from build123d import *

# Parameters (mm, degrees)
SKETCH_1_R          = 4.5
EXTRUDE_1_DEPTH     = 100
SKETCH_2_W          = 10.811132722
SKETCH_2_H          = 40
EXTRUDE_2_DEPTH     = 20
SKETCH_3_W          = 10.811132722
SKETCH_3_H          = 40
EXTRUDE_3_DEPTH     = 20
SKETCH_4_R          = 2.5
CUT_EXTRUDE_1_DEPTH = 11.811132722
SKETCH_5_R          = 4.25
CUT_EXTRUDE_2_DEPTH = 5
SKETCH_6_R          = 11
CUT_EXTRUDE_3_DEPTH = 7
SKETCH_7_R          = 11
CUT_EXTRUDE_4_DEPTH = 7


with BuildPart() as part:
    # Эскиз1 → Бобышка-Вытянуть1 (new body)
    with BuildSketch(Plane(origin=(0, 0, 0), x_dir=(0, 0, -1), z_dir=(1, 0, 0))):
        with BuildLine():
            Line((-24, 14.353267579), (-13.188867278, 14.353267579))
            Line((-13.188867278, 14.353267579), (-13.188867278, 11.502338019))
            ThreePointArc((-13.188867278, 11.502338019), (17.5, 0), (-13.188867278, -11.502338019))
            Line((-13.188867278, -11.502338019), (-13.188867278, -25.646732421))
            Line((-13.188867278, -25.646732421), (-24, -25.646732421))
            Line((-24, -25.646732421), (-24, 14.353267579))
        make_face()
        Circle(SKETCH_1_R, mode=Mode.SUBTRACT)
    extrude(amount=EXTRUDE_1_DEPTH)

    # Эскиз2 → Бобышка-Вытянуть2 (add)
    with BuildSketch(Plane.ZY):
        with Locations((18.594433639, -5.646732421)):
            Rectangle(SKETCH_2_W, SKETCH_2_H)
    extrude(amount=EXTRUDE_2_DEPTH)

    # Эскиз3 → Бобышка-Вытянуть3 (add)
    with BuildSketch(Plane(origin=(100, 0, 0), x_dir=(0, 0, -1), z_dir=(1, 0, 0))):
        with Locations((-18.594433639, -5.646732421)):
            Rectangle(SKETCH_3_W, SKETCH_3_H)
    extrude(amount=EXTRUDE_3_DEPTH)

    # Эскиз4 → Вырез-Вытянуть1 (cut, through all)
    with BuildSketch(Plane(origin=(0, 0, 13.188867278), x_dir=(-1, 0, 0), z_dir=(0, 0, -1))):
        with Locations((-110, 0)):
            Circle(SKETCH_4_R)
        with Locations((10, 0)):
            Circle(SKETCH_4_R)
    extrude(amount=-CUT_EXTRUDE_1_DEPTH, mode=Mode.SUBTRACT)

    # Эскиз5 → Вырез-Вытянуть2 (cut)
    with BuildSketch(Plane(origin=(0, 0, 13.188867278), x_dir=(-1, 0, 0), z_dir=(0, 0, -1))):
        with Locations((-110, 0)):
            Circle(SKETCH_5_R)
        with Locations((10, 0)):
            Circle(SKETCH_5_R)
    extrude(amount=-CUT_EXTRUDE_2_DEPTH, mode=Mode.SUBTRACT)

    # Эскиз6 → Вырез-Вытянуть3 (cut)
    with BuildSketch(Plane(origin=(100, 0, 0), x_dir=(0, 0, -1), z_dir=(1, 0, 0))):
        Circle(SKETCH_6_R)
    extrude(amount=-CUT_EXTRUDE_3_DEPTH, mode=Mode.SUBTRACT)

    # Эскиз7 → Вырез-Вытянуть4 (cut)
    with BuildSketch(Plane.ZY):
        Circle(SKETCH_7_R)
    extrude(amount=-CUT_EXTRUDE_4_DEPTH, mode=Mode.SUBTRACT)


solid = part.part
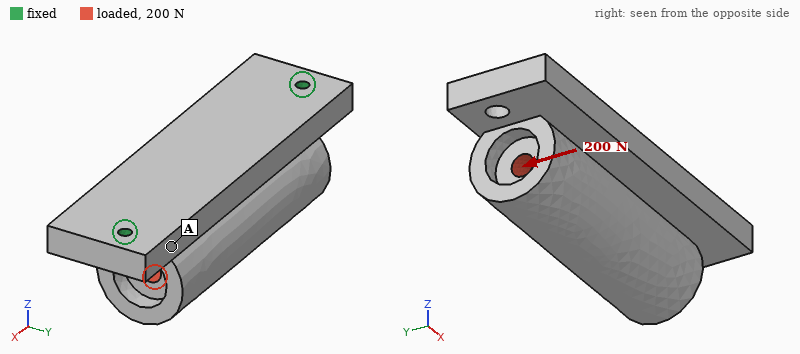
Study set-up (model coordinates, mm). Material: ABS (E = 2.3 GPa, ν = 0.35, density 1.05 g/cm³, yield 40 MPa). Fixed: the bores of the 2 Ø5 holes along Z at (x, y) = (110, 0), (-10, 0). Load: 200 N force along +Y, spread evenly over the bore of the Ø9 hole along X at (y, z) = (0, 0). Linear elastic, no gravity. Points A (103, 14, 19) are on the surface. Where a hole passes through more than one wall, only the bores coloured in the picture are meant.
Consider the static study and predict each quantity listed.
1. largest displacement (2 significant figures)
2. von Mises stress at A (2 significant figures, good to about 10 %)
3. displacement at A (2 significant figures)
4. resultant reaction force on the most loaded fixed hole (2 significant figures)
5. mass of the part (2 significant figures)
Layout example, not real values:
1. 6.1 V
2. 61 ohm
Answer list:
1. 0.34 mm
2. 2.1 MPa
3. 0.098 mm
4. 110 N
5. 150 g
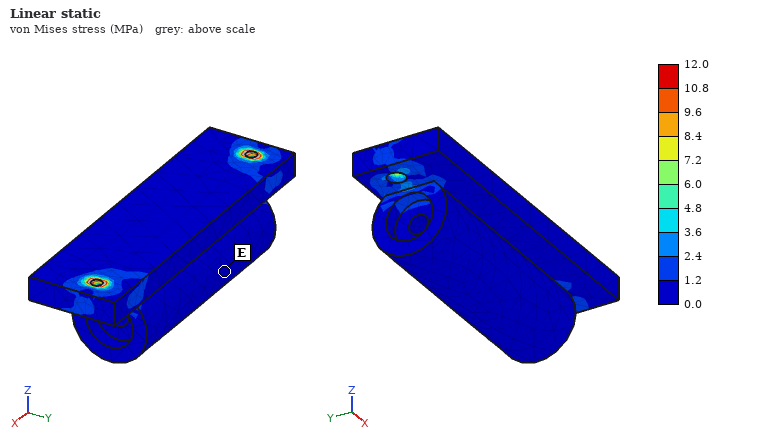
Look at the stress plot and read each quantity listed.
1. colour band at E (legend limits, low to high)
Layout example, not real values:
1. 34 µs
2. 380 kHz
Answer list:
1. 0.0 to 1.2 MPa
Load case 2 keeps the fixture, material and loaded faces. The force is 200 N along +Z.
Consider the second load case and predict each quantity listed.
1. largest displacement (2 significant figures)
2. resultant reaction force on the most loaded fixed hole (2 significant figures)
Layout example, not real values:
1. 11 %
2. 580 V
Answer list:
1. 31 µm
2. 140 N
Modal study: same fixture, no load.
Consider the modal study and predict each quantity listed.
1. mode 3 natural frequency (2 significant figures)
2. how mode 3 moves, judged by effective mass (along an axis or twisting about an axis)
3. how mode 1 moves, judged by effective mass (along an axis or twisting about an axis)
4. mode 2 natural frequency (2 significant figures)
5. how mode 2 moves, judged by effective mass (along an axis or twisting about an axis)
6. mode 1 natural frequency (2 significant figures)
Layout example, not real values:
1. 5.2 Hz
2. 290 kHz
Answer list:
1. 1700 Hz
2. along Y
3. along Y
4. 1200 Hz
5. along Z
6. 440 Hz
